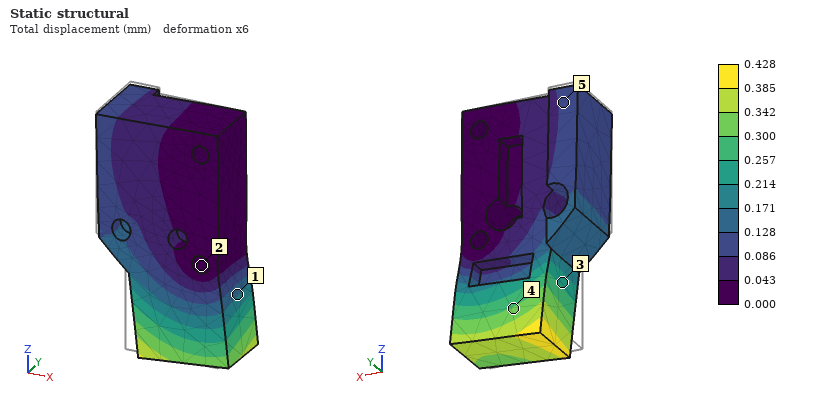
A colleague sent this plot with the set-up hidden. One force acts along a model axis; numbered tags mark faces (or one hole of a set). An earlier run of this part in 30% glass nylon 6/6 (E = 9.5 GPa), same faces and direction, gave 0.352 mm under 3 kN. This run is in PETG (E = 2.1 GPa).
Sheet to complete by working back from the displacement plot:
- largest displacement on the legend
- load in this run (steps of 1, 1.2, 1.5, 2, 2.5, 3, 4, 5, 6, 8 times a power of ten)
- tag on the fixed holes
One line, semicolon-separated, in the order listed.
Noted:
0.428 mm; 800 N; 2
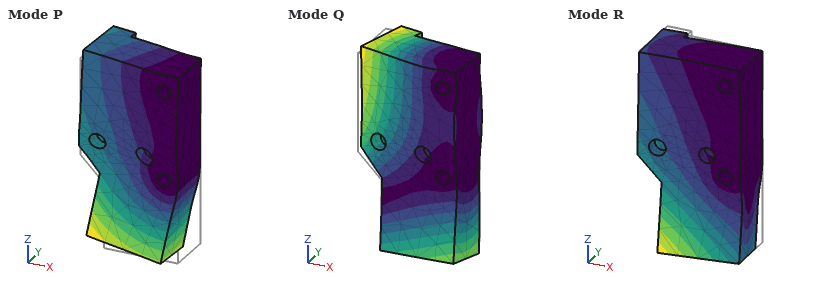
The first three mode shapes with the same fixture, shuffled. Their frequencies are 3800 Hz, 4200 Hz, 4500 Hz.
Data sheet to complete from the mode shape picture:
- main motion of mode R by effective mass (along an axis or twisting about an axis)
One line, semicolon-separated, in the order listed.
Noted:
along Y
